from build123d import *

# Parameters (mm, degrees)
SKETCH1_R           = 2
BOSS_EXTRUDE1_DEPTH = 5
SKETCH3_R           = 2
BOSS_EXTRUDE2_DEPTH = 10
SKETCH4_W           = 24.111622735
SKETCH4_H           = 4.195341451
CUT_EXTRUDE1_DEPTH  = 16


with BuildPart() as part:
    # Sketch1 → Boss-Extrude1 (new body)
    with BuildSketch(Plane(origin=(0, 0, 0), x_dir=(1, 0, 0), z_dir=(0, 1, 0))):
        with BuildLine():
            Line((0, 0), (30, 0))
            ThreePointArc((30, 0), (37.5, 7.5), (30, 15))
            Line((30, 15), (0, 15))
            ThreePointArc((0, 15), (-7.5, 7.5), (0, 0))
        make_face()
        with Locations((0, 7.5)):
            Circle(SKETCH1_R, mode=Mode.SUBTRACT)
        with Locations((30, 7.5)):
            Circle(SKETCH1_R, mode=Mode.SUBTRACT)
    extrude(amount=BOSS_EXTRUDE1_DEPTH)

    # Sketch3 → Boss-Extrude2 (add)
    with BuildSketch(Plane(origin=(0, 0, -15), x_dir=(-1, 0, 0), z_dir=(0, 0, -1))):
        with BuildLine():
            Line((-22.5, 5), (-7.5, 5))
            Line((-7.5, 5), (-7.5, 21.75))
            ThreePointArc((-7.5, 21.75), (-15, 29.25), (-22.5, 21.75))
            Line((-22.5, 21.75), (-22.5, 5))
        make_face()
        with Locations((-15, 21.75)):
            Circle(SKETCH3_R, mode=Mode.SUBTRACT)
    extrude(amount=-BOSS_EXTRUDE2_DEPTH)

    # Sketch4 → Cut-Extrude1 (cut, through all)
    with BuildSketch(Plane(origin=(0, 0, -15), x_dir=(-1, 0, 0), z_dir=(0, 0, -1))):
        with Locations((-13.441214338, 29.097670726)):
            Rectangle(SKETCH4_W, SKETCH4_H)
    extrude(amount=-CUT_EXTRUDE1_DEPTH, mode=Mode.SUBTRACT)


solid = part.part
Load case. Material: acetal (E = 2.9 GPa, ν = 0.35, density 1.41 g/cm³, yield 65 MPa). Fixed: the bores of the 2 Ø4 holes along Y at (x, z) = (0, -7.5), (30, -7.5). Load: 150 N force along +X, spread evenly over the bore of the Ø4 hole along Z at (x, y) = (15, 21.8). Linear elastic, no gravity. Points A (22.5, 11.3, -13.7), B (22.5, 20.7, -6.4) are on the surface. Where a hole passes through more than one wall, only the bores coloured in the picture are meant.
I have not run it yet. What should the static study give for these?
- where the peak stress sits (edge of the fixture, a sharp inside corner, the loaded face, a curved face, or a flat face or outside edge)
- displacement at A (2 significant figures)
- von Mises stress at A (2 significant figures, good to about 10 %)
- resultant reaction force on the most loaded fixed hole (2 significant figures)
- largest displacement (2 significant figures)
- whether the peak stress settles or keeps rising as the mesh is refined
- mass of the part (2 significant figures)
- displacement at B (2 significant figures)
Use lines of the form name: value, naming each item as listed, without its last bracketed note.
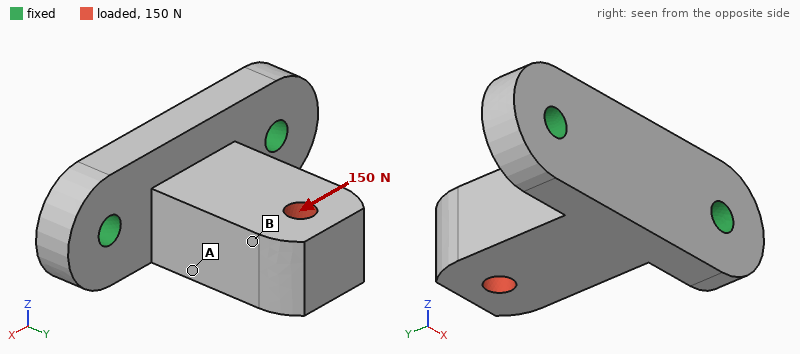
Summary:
where the peak stress sits: edge of the fixture
displacement at A: 0.063 mm
von Mises stress at A: 3.7 MPa
resultant reaction force on the most loaded fixed hole: 150 N
largest displacement: 0.17 mm
whether the peak stress settles or keeps rising as the mesh is refined: keeps rising
mass of the part: 8.6 g
displacement at B: 0.13 mm
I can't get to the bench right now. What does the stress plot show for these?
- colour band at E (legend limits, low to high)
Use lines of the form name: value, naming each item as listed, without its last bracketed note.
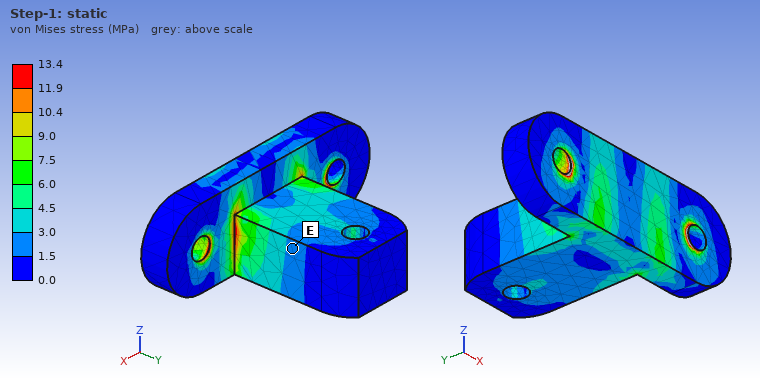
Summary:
colour band at E: 1.5 to 3.0 MPa
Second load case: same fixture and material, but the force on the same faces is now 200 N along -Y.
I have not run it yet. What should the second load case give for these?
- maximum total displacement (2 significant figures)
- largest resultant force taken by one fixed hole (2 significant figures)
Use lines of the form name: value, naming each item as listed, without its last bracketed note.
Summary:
maximum total displacement: 0.10 mm
largest resultant force taken by one fixed hole: 100 N
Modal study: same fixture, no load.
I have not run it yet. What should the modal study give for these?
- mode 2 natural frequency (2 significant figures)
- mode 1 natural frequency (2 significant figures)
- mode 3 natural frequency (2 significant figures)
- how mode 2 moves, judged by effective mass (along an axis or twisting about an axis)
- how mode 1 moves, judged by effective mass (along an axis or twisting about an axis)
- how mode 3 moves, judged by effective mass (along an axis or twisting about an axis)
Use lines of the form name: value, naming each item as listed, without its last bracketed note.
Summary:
mode 2 natural frequency: 3500 Hz
mode 1 natural frequency: 1700 Hz
mode 3 natural frequency: 4800 Hz
how mode 2 moves, judged by effective mass: along X
how mode 1 moves, judged by effective mass: along Z
how mode 3 moves, judged by effective mass: along Y
